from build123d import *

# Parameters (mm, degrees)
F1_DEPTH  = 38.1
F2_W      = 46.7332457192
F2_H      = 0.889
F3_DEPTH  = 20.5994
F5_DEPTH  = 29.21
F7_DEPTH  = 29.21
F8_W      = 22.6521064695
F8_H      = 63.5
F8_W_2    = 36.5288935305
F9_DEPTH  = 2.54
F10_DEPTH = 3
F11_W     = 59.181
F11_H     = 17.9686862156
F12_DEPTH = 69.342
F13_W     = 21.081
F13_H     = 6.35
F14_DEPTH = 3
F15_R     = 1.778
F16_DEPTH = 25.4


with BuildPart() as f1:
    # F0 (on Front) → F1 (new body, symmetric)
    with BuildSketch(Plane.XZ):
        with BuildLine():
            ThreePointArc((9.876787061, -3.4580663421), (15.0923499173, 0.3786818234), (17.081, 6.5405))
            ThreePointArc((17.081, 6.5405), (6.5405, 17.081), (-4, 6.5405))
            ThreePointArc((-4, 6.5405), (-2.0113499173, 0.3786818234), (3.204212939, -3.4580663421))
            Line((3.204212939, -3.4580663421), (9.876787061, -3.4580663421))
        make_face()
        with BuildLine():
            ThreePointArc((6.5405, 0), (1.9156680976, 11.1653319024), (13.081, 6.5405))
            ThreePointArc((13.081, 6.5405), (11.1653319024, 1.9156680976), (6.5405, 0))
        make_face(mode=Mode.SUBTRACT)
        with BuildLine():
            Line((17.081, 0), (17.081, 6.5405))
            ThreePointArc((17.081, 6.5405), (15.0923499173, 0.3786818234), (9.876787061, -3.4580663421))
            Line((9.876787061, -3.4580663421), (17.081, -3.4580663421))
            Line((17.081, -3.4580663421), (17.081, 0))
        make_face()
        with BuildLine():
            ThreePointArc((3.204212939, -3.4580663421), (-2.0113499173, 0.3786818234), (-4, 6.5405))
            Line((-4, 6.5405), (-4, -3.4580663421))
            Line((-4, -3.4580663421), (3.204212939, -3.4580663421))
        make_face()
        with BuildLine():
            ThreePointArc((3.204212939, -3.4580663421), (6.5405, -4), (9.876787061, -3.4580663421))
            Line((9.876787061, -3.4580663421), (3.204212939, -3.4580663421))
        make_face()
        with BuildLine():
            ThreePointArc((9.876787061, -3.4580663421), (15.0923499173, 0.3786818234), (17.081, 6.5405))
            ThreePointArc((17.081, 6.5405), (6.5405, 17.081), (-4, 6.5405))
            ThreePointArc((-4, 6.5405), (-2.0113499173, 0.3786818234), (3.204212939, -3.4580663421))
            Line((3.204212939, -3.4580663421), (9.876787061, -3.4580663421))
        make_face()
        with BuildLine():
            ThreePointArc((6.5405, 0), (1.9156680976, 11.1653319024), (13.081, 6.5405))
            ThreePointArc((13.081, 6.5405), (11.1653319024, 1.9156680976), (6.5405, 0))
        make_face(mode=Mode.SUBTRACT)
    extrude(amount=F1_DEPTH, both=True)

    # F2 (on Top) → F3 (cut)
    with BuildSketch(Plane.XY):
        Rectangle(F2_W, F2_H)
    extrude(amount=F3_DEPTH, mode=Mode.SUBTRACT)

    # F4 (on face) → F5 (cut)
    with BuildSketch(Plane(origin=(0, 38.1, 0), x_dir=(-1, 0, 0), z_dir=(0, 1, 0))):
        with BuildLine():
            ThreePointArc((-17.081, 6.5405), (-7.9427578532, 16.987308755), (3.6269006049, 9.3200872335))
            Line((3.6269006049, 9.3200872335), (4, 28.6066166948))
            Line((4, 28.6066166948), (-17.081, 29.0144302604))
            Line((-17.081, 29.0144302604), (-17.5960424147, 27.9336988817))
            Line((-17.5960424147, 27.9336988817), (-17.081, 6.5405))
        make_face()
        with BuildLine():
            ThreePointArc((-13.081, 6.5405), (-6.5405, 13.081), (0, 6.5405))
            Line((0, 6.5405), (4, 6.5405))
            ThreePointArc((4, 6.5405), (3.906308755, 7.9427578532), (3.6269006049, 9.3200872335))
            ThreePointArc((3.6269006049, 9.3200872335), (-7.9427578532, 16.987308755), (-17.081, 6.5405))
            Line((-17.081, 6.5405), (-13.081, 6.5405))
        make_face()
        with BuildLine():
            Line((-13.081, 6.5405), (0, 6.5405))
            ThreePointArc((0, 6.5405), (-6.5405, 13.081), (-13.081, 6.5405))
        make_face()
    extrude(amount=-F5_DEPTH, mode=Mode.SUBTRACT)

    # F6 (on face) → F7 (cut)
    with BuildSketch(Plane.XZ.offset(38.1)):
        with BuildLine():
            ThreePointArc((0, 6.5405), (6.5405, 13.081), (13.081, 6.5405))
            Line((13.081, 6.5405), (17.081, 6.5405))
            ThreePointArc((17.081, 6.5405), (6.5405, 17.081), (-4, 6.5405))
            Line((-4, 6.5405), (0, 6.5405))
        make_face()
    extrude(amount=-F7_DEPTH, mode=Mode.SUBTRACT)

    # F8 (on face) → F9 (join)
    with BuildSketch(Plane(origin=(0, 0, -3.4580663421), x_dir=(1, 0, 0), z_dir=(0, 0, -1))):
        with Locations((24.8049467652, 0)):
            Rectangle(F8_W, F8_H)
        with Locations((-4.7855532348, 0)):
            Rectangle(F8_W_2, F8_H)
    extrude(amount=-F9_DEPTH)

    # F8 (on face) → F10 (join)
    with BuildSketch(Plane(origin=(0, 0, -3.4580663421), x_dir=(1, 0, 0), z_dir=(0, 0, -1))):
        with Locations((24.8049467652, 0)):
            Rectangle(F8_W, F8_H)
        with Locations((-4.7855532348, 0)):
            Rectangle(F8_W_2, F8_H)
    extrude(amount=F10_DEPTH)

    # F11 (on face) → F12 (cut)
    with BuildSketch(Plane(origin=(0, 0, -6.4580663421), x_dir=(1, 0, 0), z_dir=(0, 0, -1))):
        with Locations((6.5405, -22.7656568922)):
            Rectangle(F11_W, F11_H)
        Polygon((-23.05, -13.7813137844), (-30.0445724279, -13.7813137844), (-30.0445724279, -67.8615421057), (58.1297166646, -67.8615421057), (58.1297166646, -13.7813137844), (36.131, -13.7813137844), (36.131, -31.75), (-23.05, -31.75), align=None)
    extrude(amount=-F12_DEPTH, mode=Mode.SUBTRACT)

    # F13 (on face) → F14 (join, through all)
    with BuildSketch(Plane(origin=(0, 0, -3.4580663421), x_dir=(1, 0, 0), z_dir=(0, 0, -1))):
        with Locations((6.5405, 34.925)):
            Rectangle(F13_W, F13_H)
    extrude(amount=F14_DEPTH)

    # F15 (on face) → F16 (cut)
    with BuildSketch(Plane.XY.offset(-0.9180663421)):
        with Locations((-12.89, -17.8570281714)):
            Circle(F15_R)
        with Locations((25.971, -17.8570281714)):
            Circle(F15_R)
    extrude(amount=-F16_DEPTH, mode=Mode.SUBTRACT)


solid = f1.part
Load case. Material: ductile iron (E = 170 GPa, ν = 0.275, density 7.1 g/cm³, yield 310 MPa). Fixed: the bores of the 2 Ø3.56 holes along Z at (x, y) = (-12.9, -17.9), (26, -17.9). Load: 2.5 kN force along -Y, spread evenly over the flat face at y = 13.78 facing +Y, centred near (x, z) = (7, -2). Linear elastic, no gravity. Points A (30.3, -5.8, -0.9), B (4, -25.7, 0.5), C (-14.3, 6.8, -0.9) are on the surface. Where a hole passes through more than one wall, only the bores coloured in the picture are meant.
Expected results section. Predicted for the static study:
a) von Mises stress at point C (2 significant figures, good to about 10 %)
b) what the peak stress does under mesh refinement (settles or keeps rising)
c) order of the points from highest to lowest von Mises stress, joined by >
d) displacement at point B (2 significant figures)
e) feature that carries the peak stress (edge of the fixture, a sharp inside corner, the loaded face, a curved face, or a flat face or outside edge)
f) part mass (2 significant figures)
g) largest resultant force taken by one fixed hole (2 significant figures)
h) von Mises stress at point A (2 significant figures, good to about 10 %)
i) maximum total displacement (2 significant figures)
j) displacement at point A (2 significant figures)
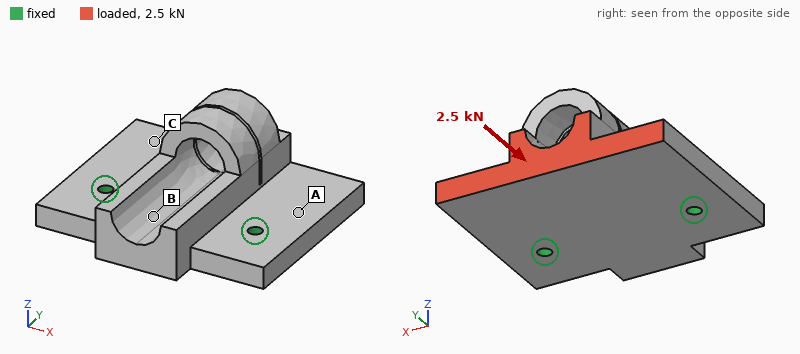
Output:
8.2 MPa
keeps rising
A > C > B
2.1 µm
edge of the fixture
160 g
1.3 kN
12 MPa
11 µm
2.0 µm
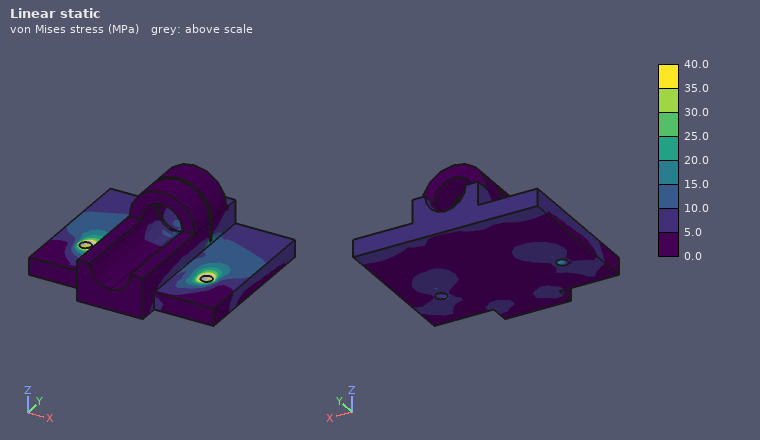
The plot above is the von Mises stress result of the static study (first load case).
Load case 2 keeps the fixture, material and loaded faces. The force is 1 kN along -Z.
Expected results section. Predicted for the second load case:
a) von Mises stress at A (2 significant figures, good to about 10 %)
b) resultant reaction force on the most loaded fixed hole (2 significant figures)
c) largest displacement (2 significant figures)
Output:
43 MPa
550 N
80 µm
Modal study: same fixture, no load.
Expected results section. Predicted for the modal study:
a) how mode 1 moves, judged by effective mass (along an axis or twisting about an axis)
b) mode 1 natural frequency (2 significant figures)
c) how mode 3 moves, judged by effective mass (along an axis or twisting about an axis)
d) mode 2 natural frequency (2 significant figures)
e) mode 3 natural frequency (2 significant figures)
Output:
along Z
3100 Hz
along Z
6900 Hz
9400 Hz
